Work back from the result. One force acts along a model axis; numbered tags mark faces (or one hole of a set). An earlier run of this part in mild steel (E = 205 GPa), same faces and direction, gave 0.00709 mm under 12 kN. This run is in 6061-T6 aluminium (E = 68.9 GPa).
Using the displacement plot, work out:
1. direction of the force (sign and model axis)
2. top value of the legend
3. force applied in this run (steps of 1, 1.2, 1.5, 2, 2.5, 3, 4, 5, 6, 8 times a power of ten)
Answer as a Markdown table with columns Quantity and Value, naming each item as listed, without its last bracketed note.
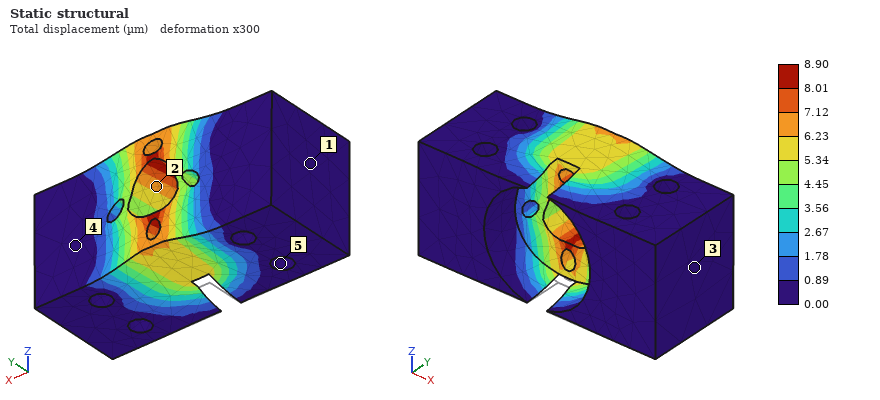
| Quantity | Value |
|---|---|
| direction of the force | +Z |
| top value of the legend | 8.90 µm |
| force applied in this run | 5 kN |
